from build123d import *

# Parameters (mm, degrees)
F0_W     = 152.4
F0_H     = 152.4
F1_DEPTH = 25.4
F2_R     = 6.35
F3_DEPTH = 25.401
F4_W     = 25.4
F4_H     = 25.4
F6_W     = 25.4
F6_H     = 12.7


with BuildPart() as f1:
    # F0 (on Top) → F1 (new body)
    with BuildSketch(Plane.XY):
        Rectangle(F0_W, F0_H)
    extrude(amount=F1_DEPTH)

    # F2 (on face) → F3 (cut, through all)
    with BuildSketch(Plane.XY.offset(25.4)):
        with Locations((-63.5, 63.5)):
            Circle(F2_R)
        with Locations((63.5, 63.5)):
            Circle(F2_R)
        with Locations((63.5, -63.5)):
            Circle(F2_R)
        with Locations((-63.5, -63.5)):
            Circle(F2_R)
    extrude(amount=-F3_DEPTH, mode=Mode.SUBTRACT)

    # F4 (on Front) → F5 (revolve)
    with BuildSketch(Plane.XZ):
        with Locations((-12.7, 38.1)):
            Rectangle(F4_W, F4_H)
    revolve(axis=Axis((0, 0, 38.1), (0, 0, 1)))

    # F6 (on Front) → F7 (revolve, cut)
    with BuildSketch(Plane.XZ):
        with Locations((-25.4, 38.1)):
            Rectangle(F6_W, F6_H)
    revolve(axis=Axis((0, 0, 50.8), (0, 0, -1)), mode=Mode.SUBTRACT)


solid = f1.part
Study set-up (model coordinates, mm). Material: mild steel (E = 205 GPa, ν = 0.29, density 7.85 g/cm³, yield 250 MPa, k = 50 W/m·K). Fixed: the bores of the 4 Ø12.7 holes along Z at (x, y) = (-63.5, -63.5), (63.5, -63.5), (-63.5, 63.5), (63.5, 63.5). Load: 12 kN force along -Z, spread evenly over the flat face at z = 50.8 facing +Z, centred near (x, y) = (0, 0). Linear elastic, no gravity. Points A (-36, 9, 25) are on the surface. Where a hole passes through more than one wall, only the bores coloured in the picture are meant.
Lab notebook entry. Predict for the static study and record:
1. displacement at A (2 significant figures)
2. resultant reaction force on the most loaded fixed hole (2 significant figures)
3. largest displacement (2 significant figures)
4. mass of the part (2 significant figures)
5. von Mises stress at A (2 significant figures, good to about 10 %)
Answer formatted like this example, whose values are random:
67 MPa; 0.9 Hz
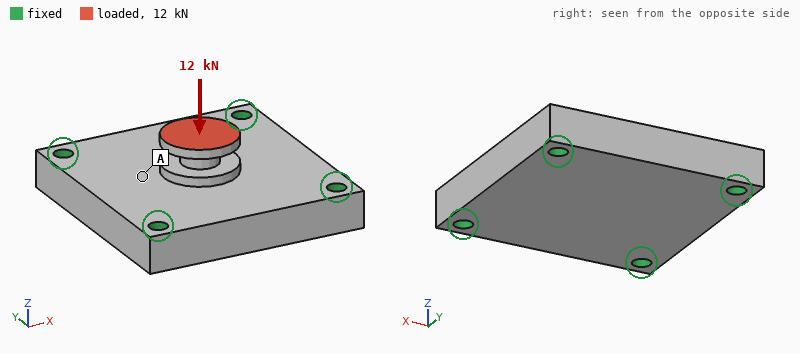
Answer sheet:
6.5 µm; 3.0 kN; 22 µm; 4.8 kg; 8.2 MPa
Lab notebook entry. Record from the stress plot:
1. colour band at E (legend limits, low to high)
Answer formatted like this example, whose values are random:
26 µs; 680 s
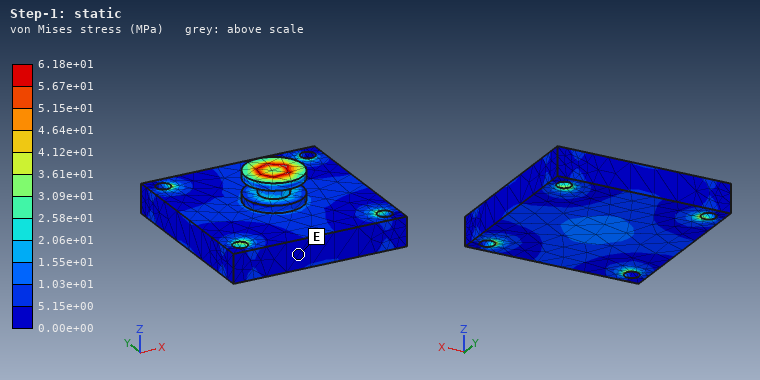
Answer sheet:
0.00e+00 to 5.15e+00 MPa
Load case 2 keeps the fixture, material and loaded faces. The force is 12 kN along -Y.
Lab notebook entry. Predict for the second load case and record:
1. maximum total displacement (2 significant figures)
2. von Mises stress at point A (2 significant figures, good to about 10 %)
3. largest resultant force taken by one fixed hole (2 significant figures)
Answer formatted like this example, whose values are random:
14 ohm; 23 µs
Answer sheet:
43 µm; 9.3 MPa; 4.0 kN
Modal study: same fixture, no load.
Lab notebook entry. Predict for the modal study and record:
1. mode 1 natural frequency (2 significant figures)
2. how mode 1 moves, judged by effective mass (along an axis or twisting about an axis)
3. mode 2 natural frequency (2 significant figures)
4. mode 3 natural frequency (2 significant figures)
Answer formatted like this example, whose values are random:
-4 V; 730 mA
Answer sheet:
4400 Hz; along Z; 7000 Hz; 7000 Hz
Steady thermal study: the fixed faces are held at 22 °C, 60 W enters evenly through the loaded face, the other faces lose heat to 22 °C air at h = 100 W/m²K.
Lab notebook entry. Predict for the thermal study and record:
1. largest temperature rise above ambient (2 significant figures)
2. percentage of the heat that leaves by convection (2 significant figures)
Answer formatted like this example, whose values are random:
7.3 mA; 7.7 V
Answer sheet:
56 K; 60 %
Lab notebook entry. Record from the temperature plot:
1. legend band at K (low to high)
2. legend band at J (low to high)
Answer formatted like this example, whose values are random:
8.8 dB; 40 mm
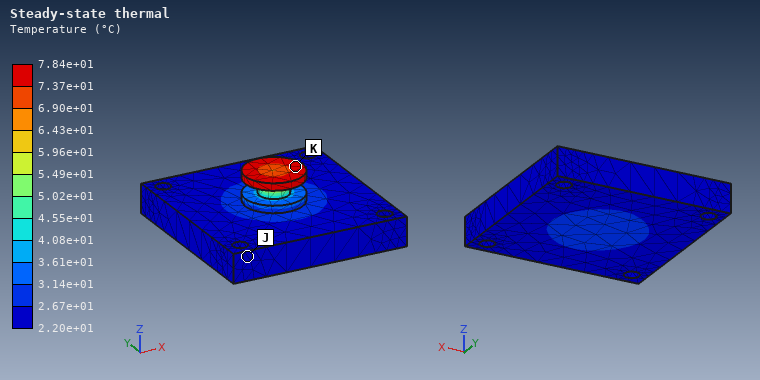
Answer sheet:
7.37e+01 to 7.84e+01 °C; 2.20e+01 to 2.67e+01 °C
